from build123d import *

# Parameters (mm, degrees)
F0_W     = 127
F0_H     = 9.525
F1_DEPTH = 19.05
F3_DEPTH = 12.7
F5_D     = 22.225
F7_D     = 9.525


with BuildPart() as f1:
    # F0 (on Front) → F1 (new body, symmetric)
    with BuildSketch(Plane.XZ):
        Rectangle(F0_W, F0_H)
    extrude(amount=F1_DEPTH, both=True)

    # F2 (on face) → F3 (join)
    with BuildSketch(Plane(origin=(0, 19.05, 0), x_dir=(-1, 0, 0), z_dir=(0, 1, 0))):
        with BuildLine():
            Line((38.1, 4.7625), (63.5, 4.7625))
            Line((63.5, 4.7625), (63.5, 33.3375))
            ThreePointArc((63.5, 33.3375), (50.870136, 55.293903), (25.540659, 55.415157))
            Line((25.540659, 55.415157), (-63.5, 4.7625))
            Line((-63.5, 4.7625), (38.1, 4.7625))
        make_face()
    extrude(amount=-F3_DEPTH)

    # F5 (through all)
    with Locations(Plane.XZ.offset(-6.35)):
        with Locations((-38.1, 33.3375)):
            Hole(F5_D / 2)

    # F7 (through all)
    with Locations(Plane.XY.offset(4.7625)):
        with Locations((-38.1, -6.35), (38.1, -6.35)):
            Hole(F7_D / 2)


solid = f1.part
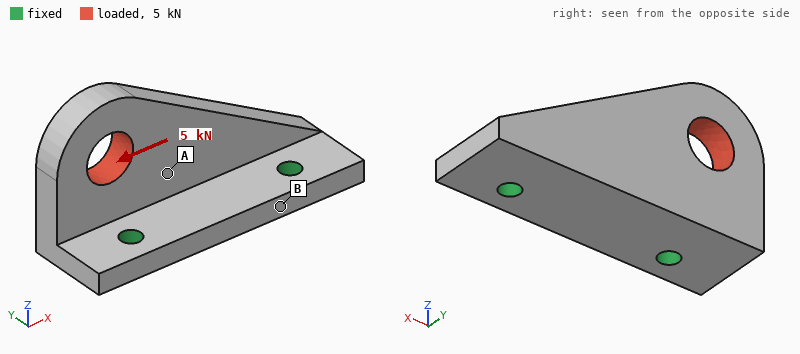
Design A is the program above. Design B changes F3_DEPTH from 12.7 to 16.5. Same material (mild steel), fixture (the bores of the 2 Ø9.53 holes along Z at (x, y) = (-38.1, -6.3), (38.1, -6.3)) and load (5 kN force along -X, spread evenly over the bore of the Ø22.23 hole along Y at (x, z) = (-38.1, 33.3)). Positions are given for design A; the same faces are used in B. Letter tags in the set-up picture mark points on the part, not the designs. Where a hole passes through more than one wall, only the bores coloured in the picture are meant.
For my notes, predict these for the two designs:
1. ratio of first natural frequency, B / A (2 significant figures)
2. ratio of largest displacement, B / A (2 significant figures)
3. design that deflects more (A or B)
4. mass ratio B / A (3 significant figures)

1.0
0.67
A
1.15
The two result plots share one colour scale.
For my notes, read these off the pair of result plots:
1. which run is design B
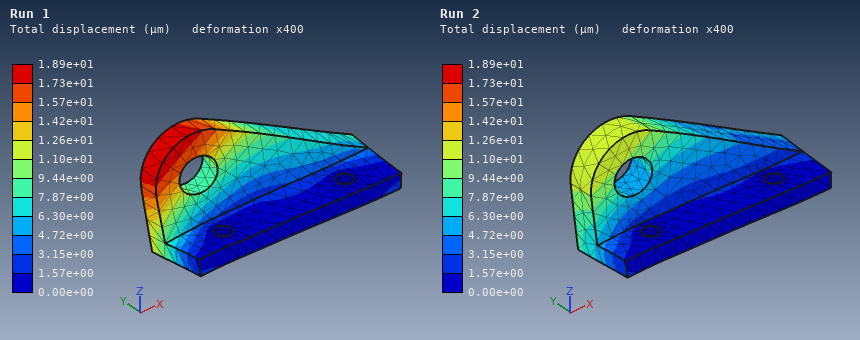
Run 2
